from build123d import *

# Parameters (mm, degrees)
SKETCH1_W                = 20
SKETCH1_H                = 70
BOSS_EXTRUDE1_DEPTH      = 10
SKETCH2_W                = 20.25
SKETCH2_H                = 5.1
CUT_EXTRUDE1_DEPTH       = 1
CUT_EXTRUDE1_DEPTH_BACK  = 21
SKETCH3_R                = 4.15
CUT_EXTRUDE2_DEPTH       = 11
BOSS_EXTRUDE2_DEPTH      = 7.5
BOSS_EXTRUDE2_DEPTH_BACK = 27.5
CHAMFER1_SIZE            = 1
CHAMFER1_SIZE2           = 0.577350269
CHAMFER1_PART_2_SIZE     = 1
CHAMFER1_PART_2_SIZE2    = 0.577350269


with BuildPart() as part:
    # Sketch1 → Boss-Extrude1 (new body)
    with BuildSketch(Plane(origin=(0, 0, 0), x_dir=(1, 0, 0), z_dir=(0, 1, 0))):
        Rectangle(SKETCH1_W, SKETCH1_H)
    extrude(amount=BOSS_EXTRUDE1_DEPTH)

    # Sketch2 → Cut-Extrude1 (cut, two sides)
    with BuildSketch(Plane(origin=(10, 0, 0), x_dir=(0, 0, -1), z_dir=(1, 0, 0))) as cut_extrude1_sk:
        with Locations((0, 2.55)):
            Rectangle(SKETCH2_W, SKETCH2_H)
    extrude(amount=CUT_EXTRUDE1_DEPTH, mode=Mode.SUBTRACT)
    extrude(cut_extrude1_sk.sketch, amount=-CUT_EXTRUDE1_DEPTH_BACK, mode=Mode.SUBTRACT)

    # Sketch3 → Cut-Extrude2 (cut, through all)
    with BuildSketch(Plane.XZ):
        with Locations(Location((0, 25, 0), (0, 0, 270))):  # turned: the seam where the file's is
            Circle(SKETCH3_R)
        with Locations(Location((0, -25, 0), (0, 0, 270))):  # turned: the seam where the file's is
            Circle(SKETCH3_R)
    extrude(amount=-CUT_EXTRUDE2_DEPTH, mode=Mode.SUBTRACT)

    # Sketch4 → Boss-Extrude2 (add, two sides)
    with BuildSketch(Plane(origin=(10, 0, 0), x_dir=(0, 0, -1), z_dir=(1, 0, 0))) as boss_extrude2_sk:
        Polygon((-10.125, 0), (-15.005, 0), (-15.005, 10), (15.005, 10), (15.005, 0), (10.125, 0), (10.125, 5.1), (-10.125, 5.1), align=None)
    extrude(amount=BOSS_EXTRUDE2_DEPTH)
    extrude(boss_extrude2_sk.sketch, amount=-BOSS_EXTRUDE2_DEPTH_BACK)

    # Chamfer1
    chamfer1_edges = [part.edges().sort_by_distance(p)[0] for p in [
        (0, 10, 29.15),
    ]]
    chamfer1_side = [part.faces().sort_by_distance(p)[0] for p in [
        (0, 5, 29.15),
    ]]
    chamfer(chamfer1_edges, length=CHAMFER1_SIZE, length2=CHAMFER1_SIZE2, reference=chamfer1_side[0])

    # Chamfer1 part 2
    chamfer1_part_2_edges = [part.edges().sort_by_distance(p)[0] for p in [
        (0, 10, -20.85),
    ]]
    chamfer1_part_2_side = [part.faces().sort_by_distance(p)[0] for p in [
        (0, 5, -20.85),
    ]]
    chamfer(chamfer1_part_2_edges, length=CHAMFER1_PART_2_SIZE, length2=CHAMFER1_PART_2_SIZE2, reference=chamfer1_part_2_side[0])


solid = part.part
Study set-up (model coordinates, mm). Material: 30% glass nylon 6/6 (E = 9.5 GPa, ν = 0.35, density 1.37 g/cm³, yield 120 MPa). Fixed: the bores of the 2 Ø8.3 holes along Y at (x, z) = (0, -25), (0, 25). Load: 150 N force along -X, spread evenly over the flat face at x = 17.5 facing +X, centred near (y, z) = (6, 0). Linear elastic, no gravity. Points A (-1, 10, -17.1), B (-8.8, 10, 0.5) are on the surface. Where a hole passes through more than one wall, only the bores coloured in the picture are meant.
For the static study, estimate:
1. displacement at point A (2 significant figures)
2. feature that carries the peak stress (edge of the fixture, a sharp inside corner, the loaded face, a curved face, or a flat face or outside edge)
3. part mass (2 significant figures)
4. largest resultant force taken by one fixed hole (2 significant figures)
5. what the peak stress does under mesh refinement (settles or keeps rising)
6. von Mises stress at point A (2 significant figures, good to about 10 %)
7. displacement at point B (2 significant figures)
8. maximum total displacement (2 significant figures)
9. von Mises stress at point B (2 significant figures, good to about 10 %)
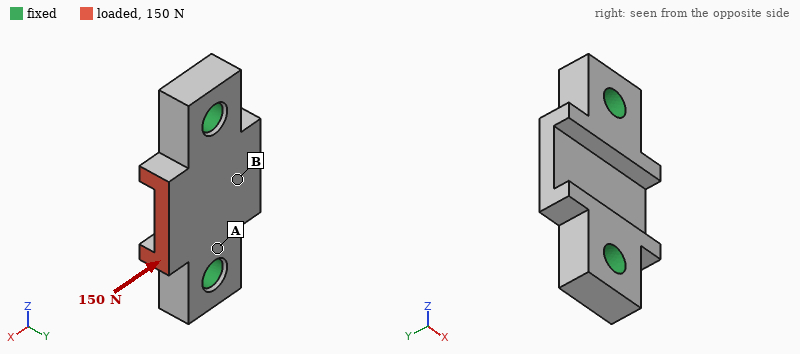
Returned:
1.1 µm
edge of the fixture
19 g
76 N
keeps rising
1.1 MPa
2.7 µm
4.6 µm
0.35 MPa
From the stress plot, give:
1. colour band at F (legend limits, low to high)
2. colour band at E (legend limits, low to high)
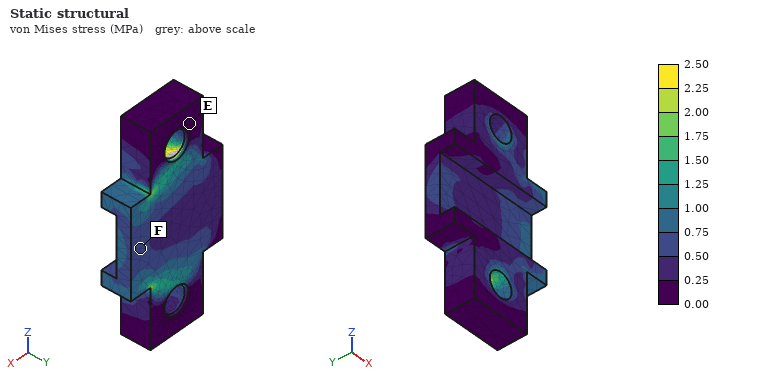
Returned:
0.50 to 0.75 MPa
0.00 to 0.25 MPa
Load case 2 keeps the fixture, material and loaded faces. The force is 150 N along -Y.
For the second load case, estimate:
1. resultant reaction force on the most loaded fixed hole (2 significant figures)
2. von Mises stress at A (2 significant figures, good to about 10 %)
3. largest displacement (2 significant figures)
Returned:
88 N
3.3 MPa
42 µm
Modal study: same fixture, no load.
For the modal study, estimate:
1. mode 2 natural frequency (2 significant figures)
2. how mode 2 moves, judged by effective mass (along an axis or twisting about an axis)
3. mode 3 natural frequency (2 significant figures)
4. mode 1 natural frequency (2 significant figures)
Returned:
8400 Hz
along Y
13 kHz
7700 Hz
